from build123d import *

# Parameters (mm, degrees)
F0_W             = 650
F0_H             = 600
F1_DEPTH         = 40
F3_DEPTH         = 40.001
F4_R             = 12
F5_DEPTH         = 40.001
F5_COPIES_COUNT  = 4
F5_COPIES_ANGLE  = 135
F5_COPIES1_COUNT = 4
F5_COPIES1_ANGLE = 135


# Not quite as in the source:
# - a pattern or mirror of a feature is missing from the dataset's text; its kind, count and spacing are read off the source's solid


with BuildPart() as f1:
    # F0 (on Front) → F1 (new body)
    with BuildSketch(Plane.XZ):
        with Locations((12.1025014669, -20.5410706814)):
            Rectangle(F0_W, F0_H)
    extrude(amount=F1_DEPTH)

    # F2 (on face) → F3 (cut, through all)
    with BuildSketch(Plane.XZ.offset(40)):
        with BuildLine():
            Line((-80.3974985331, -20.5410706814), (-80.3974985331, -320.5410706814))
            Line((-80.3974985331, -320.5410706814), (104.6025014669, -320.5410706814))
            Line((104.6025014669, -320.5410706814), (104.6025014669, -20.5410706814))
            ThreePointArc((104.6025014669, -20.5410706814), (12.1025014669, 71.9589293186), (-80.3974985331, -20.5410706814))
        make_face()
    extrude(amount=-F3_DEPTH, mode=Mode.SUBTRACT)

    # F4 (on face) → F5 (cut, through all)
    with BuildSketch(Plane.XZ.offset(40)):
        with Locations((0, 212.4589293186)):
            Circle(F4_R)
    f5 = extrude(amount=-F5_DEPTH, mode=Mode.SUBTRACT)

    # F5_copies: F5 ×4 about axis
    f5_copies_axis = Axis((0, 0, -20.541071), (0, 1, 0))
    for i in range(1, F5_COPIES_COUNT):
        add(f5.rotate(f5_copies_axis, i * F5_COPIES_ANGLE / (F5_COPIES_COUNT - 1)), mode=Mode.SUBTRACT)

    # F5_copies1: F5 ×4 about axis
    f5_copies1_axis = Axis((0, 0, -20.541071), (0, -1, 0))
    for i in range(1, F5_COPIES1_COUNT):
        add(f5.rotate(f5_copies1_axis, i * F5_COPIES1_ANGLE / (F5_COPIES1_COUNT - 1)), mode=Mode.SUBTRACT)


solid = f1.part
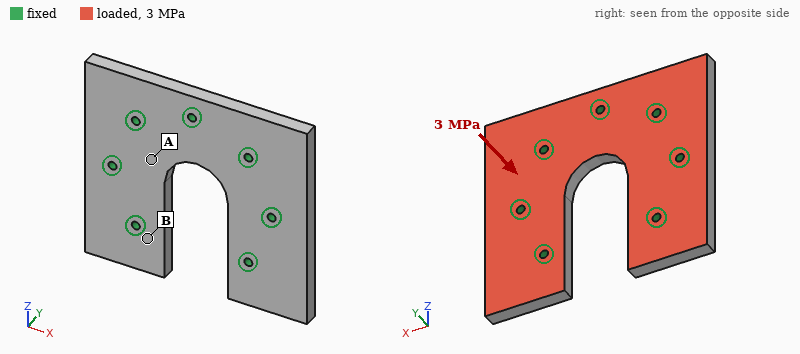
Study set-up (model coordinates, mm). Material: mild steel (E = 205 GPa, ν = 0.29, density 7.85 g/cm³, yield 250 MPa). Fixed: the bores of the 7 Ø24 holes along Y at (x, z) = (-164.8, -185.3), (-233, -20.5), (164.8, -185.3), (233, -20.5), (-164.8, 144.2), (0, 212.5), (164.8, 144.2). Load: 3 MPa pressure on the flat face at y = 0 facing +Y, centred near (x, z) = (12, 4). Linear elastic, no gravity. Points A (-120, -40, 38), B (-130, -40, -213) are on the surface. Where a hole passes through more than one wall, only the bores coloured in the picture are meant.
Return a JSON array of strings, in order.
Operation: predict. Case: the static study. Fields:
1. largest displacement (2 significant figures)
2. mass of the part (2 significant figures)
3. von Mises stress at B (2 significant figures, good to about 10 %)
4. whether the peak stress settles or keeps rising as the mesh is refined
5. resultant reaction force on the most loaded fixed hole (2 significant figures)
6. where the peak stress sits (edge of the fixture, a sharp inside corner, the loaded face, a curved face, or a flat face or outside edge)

["0.53 mm", "100 kg", "73 MPa", "keeps rising", "170 kN", "edge of the fixture"]
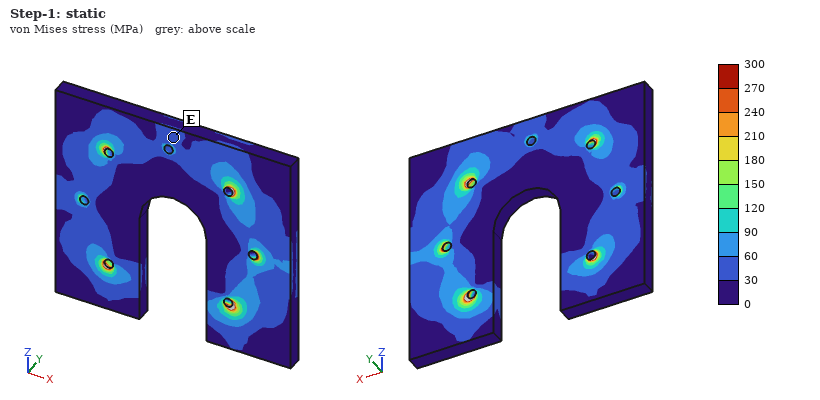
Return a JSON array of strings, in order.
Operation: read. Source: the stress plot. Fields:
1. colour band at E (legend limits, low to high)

["30 to 60 MPa"]
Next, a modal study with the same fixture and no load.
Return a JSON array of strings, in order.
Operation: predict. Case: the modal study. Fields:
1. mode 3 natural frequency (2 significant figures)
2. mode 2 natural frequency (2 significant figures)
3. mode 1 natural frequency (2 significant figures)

["1100 Hz", "1000 Hz", "940 Hz"]
